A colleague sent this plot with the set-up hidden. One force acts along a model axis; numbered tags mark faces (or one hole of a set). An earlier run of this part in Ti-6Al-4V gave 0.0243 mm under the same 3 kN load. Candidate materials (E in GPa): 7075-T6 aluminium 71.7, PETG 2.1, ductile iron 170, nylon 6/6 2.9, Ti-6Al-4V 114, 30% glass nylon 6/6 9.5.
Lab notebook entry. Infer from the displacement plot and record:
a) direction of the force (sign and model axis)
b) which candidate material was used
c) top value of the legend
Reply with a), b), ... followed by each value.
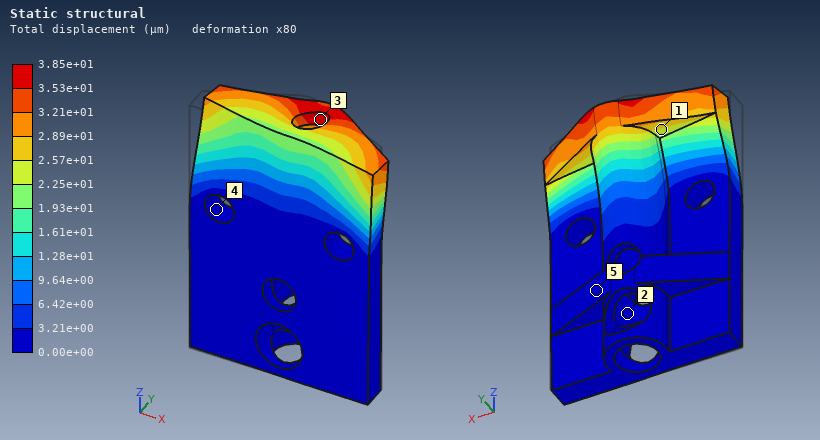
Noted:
a) +X
b) 7075-T6 aluminium
c) 3.85e+01 µm
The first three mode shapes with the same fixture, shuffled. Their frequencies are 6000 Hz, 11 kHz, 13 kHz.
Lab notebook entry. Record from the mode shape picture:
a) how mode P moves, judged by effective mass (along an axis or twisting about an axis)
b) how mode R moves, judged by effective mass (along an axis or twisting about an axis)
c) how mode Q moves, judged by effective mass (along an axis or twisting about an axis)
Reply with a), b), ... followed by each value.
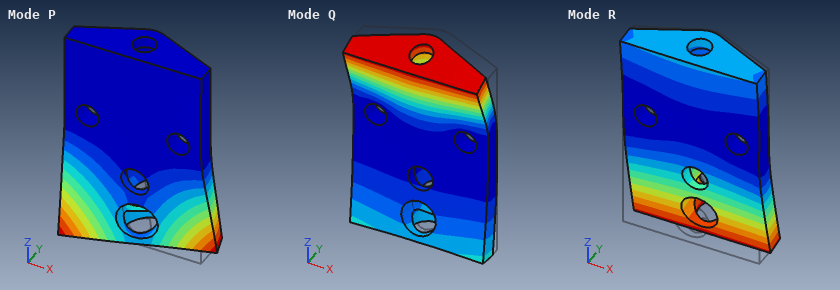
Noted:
a) twisting about Z
b) along Y
c) along Y
